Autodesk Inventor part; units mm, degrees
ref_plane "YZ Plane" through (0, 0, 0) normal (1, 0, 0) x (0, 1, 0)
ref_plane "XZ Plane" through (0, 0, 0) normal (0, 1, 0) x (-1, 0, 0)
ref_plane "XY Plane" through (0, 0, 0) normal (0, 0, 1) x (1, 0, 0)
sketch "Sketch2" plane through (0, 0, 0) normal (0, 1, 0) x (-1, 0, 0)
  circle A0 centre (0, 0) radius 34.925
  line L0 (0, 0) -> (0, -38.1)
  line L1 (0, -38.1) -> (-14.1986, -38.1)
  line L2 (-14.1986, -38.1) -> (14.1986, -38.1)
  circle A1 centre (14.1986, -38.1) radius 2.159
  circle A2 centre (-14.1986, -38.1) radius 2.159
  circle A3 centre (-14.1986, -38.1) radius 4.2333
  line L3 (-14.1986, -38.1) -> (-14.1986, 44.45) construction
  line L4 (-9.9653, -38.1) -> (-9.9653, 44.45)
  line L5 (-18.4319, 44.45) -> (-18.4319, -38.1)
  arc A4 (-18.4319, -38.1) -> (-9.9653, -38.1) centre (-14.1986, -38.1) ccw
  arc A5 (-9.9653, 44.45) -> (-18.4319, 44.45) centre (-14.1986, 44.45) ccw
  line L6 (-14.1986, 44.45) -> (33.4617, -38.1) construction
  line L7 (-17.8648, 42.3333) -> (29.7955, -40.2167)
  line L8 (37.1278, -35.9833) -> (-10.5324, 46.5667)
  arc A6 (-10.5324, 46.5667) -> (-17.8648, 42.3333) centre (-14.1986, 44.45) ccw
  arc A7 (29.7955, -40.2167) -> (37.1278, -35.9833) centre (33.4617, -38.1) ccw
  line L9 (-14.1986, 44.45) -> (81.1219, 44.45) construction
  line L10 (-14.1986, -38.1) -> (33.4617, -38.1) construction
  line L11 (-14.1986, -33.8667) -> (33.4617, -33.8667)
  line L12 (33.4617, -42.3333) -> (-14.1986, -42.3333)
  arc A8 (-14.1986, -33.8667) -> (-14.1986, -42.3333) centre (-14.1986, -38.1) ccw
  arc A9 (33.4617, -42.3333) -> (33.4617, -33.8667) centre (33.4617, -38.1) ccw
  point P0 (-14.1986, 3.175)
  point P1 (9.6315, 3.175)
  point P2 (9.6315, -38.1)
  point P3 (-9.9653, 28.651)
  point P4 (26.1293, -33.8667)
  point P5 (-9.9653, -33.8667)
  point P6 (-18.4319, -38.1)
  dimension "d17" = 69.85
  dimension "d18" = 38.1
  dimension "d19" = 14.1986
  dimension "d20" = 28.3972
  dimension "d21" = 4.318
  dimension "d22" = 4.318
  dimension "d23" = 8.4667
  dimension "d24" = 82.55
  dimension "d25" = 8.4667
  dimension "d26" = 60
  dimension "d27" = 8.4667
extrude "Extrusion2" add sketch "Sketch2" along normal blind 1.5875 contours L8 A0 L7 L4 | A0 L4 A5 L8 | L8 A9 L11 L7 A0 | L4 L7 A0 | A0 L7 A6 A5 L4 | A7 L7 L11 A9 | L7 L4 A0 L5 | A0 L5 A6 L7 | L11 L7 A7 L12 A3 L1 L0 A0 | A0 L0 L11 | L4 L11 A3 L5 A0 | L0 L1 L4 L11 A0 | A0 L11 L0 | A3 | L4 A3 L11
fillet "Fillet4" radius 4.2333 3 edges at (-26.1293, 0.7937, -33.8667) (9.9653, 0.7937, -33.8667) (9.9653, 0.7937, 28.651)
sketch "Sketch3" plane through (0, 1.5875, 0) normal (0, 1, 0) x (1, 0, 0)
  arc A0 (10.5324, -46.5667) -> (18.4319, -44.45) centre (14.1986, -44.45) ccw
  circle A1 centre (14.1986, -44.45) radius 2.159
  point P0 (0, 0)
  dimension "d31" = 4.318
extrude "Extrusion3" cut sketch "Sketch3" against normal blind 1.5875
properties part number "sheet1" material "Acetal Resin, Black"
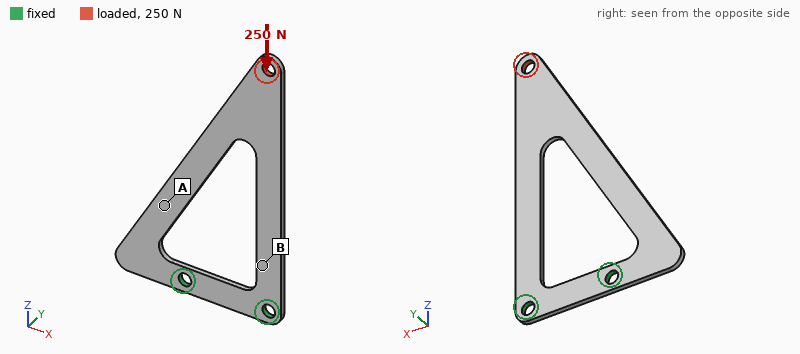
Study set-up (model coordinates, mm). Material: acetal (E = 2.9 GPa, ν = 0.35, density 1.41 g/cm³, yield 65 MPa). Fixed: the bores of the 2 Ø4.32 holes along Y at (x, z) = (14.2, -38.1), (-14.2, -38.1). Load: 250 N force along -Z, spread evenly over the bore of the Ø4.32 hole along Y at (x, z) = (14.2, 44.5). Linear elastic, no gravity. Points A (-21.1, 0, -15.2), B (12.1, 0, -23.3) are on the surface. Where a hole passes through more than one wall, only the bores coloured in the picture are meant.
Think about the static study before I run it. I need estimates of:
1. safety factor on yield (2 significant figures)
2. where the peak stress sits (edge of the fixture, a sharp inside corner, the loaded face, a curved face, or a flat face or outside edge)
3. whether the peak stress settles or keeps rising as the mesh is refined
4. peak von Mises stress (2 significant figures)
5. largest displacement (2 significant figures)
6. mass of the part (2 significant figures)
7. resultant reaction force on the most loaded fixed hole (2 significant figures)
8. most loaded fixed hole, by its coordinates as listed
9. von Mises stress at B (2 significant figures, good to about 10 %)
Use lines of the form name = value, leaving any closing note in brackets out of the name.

safety factor on yield = 1.2
where the peak stress sits = the loaded face
whether the peak stress settles or keeps rising as the mesh is refined = settles
peak von Mises stress = 55 MPa
largest displacement = 1.1 mm
mass of the part = 4.2 g
resultant reaction force on the most loaded fixed hole = 250 N
most loaded fixed hole, by its coordinates as listed = (14.2, -38.1)
von Mises stress at B = 17 MPa
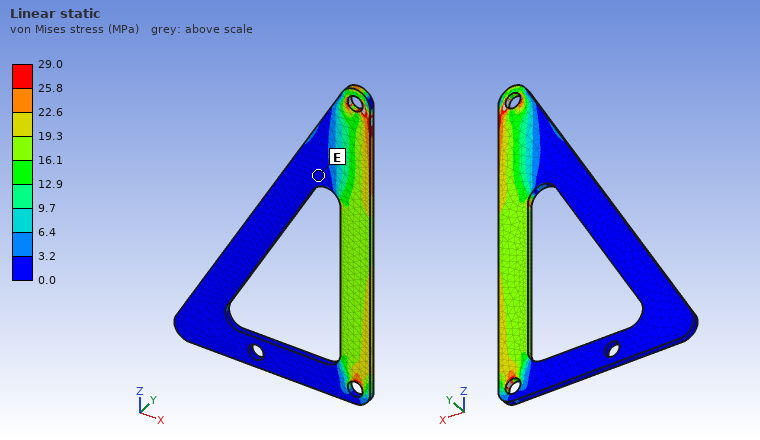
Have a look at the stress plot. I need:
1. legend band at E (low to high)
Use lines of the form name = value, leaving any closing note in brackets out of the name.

legend band at E = 0.0 to 3.2 MPa
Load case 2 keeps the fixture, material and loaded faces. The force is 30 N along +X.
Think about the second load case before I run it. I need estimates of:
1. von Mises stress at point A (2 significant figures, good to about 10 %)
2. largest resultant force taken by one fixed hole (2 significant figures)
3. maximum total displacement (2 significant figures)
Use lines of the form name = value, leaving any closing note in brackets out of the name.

von Mises stress at point A = 3.4 MPa
largest resultant force taken by one fixed hole = 65 N
maximum total displacement = 1.2 mm
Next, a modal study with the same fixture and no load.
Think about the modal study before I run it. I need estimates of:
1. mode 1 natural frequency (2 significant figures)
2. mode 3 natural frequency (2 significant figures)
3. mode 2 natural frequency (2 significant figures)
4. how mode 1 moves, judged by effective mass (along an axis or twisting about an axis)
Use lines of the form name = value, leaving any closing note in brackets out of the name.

mode 1 natural frequency = 54 Hz
mode 3 natural frequency = 380 Hz
mode 2 natural frequency = 270 Hz
how mode 1 moves, judged by effective mass = along Y
